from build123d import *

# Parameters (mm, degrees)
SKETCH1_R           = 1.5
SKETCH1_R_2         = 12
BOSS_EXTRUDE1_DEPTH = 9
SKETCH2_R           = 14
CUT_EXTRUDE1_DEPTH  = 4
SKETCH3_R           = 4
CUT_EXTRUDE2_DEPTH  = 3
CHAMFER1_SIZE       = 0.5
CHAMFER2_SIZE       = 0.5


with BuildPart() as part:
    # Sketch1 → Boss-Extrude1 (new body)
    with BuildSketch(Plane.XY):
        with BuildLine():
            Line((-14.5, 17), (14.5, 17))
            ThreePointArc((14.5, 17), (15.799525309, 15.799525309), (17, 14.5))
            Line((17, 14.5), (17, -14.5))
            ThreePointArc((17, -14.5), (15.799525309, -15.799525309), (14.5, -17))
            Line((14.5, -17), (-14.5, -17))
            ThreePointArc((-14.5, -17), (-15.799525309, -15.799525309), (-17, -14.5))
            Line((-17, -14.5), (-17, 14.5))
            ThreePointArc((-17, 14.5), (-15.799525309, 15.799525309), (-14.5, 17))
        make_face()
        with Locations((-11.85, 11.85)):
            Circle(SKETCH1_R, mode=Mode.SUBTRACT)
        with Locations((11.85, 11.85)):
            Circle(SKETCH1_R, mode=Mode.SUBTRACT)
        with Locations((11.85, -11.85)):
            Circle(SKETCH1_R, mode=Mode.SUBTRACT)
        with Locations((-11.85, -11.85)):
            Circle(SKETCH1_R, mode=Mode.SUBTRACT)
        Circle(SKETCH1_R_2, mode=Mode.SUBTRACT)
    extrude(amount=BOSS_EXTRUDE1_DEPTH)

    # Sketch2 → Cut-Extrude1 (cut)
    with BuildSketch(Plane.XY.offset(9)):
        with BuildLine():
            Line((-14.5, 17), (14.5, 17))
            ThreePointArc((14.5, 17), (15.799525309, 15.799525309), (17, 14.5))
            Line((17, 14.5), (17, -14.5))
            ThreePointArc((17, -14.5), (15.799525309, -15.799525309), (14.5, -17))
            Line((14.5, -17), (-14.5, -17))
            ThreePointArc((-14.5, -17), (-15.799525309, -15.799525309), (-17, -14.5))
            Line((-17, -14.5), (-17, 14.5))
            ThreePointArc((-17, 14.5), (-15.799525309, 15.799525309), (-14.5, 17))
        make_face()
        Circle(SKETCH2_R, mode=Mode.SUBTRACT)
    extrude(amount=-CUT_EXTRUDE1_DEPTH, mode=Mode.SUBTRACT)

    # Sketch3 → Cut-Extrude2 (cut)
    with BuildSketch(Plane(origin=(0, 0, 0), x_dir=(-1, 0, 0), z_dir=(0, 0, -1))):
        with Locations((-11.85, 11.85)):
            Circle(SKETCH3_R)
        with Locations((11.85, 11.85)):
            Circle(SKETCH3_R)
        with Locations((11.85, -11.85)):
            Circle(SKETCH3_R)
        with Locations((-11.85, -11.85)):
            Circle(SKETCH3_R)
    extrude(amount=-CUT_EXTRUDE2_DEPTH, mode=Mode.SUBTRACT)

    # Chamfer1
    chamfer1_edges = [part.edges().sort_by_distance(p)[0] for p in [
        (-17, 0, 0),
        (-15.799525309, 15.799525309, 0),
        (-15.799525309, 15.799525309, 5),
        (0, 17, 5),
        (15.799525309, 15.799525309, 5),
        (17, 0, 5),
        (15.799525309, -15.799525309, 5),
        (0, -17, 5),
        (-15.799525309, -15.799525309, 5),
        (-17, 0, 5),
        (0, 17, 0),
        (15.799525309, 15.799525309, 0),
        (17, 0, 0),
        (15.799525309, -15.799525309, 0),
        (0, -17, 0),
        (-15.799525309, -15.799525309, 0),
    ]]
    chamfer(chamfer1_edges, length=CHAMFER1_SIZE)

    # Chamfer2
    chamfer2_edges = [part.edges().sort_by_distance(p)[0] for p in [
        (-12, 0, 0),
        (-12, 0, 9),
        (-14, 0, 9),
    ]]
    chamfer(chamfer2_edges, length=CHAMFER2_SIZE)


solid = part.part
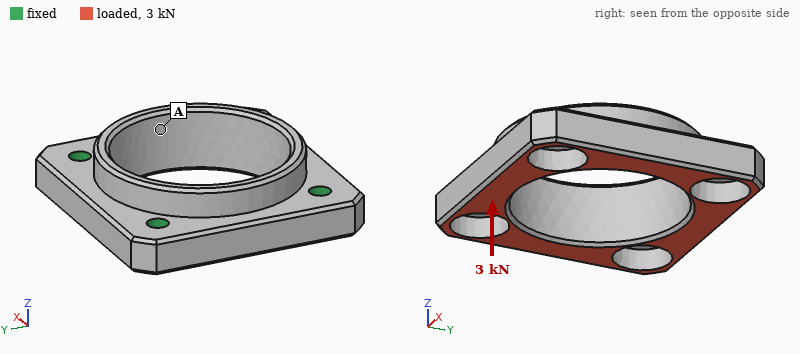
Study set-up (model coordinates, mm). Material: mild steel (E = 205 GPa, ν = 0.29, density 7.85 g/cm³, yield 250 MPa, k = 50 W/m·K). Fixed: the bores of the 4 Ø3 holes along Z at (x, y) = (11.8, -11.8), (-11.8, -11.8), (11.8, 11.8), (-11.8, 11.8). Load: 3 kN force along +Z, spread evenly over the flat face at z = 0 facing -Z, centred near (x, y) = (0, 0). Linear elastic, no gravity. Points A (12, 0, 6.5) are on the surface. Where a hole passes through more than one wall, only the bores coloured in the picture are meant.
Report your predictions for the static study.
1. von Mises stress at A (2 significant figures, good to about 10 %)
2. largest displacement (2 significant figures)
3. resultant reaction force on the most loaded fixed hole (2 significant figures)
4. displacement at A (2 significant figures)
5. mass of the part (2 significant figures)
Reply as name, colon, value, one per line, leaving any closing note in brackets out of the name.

von Mises stress at A: 22 MPa
largest displacement: 4.6 µm
resultant reaction force on the most loaded fixed hole: 760 N
displacement at A: 3.3 µm
mass of the part: 27 g
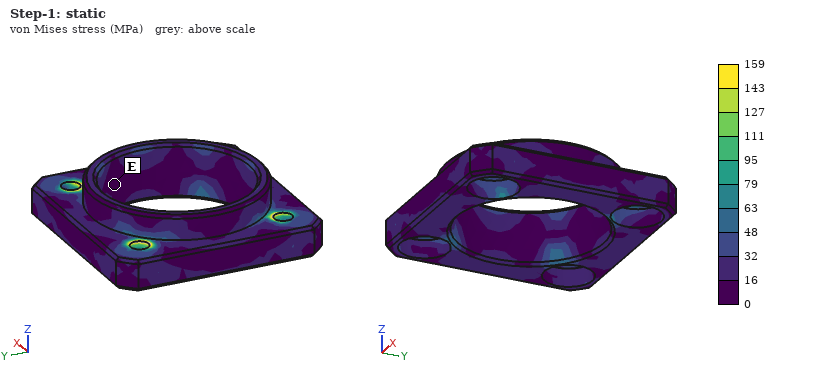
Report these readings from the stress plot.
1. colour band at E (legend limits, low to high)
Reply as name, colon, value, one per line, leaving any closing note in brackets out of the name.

colour band at E: 0 to 16 MPa
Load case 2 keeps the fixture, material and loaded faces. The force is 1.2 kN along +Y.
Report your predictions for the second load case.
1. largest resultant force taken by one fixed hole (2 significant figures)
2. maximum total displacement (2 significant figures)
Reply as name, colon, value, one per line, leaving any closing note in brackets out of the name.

largest resultant force taken by one fixed hole: 310 N
maximum total displacement: 2.9 µm
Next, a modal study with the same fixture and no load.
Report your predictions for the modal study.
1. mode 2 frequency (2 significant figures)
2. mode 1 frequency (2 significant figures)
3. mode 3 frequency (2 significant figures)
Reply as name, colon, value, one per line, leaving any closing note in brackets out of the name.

mode 2 frequency: 28 kHz
mode 1 frequency: 23 kHz
mode 3 frequency: 28 kHz
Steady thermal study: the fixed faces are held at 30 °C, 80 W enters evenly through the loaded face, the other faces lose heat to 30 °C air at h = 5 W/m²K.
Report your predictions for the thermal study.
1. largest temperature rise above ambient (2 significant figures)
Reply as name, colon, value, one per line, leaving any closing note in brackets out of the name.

largest temperature rise above ambient: 69 K
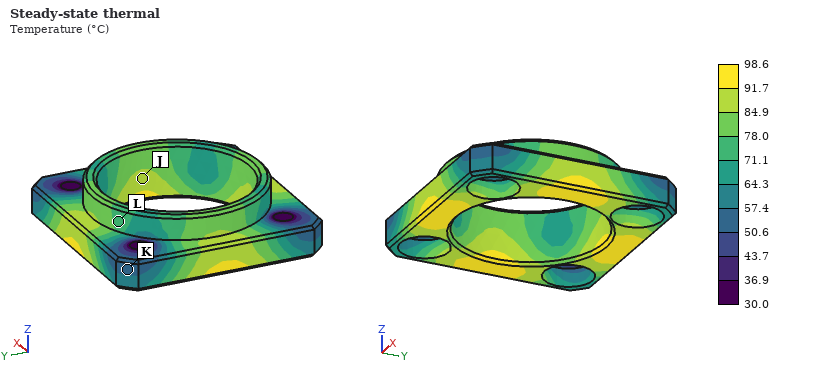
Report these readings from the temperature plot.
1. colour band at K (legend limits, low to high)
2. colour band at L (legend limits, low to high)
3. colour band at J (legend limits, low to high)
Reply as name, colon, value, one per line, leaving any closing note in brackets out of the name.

colour band at K: 50.6 to 57.4 °C
colour band at L: 71.1 to 78.0 °C
colour band at J: 84.9 to 91.7 °C
